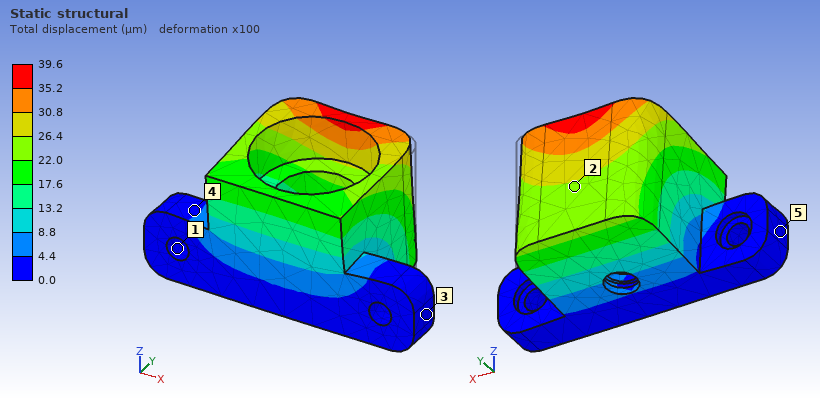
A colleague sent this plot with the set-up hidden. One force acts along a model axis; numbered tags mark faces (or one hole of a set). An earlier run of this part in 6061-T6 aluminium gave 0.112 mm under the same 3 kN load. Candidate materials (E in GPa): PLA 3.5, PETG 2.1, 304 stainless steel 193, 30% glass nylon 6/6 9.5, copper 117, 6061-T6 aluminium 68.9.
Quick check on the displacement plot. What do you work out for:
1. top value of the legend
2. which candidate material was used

39.6 µm
304 stainless steel
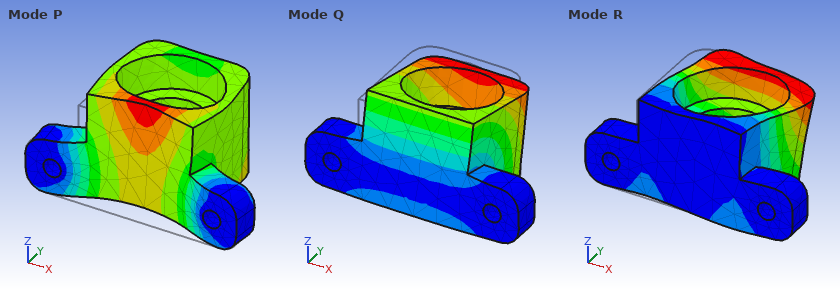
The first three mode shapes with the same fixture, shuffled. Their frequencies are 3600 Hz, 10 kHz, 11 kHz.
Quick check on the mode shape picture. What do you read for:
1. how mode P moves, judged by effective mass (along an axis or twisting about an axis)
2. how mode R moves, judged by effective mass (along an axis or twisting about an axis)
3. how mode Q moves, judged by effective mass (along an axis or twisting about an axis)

along Y
along X
along Z
